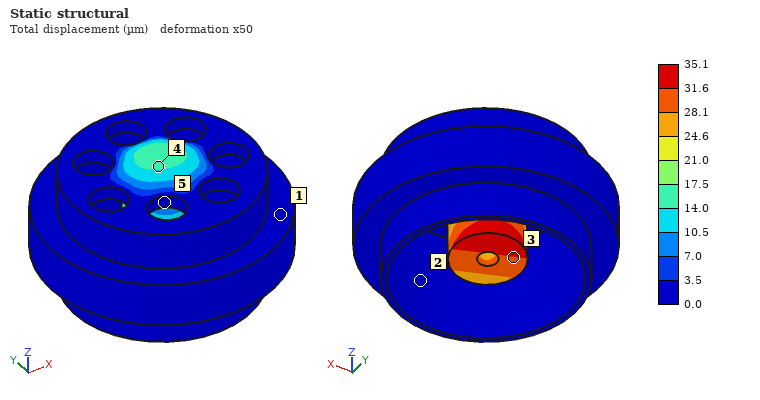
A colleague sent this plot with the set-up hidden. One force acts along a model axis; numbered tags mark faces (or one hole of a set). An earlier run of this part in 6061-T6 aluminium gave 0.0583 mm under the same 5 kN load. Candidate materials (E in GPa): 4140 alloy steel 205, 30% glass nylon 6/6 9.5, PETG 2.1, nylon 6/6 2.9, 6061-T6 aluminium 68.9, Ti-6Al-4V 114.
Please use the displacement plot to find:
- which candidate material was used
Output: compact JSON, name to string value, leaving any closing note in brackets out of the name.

{"which candidate material was used": "Ti-6Al-4V"}
